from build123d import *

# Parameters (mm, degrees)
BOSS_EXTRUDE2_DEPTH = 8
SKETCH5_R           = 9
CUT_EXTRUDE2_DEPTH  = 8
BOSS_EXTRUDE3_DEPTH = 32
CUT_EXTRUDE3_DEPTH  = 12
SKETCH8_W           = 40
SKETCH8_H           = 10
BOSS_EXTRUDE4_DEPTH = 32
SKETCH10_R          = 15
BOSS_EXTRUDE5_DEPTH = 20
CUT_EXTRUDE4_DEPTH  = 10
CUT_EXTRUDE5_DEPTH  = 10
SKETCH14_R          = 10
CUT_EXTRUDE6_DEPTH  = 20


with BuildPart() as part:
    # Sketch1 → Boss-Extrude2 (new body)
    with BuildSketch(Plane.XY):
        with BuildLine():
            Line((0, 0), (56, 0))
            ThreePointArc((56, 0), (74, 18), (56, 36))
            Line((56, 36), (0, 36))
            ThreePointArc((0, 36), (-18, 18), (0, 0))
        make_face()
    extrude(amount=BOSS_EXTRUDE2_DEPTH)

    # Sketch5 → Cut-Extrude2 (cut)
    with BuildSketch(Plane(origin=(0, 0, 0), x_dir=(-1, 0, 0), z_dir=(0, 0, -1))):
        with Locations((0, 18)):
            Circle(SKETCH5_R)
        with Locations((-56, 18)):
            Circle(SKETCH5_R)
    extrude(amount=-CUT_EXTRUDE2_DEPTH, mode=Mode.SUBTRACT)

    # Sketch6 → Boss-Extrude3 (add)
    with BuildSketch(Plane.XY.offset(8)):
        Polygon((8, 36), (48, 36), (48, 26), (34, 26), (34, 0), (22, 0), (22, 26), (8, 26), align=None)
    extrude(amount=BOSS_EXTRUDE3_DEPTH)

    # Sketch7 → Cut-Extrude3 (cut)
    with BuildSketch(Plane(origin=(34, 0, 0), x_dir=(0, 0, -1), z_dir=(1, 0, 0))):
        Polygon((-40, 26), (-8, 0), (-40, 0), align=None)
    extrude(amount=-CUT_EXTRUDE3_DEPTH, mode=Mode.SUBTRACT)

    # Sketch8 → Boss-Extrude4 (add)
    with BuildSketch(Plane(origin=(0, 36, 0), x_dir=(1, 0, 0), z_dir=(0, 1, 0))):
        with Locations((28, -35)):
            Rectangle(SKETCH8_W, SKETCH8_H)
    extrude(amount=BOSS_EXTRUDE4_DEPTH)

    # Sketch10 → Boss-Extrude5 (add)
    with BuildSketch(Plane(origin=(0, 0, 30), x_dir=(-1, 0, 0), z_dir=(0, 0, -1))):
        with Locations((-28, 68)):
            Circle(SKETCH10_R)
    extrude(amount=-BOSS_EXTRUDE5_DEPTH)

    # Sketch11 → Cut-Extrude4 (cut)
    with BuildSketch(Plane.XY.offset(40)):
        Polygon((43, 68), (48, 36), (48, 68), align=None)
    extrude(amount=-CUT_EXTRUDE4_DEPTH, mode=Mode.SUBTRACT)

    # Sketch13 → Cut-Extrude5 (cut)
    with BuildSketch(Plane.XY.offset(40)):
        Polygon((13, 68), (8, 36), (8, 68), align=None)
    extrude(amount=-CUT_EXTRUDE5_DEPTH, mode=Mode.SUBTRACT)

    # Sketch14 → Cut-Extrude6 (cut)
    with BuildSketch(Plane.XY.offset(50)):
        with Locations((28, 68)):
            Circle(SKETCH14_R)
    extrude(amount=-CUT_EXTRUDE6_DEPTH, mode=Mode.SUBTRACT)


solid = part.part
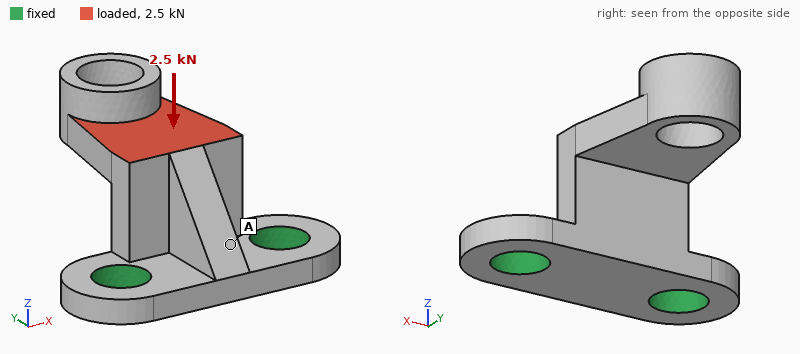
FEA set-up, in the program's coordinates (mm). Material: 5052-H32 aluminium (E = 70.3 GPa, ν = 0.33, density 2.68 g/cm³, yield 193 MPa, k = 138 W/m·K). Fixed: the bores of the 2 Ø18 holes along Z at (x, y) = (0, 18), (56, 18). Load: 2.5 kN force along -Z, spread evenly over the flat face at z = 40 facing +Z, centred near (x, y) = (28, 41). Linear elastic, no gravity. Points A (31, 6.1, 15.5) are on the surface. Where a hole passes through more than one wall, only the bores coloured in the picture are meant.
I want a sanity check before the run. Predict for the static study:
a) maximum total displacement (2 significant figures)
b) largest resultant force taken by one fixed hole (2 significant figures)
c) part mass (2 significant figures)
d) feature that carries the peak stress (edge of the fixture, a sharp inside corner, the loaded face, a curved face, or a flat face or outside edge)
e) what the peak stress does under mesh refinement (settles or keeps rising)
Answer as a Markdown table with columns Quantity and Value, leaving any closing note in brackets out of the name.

| Quantity | Value |
|---|---|
| maximum total displacement | 0.17 mm |
| largest resultant force taken by one fixed hole | 1.4 kN |
| part mass | 140 g |
| feature that carries the peak stress | edge of the fixture |
| what the peak stress does under mesh refinement | keeps rising |
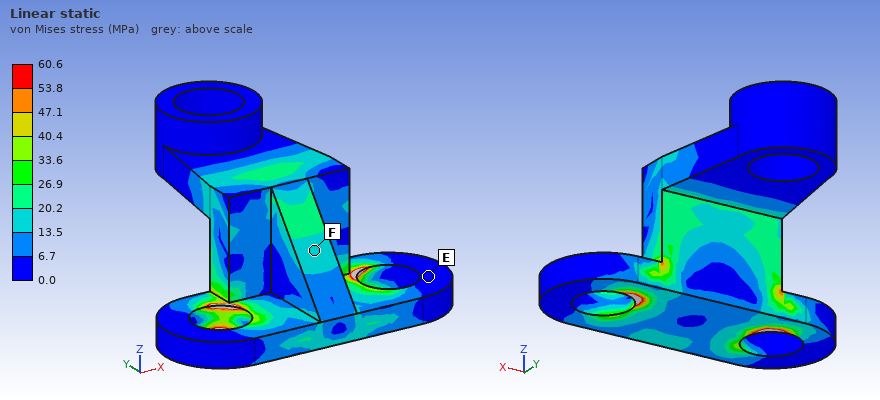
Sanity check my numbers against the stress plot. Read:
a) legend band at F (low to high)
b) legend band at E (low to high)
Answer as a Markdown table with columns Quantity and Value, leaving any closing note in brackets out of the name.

| Quantity | Value |
|---|---|
| legend band at F | 13.5 to 20.2 MPa |
| legend band at E | 0.0 to 6.7 MPa |
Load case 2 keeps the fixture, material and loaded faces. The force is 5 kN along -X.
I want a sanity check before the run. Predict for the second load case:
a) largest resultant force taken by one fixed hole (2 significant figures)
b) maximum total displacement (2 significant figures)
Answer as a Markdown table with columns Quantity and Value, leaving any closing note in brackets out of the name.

| Quantity | Value |
|---|---|
| largest resultant force taken by one fixed hole | 5.5 kN |
| maximum total displacement | 0.17 mm |
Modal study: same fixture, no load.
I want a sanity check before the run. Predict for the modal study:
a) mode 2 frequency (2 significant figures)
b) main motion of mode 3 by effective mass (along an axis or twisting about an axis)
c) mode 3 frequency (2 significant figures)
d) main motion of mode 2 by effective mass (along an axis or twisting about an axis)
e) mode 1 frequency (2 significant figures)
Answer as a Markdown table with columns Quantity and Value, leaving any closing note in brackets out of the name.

| Quantity | Value |
|---|---|
| mode 2 frequency | 3400 Hz |
| main motion of mode 3 by effective mass | along Y |
| mode 3 frequency | 5300 Hz |
| main motion of mode 2 by effective mass | along X |
| mode 1 frequency | 2100 Hz |
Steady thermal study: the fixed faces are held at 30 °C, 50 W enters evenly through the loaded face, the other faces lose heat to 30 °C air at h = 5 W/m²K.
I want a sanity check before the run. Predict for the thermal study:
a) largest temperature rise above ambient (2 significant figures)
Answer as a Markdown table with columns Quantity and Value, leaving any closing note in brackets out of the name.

| Quantity | Value |
|---|---|
| largest temperature rise above ambient | 36 K |
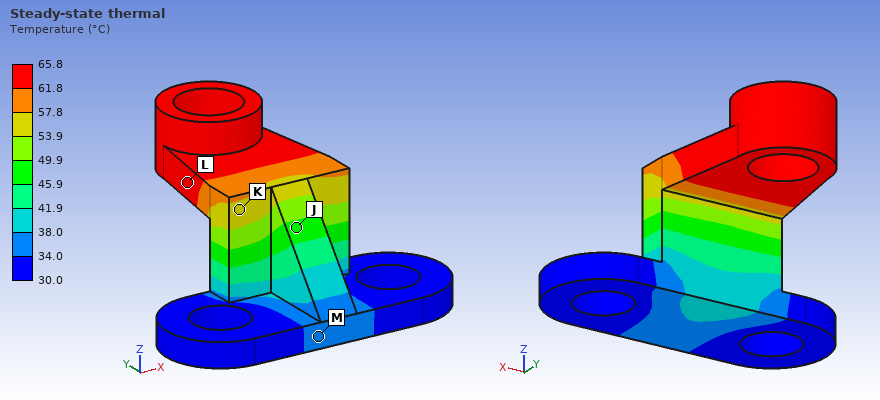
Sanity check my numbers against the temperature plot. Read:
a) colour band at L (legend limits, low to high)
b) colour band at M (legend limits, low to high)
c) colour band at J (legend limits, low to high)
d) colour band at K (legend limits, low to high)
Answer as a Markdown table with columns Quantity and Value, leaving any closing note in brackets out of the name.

| Quantity | Value |
|---|---|
| colour band at L | 61.8 to 65.8 °C |
| colour band at M | 34.0 to 38.0 °C |
| colour band at J | 45.9 to 49.9 °C |
| colour band at K | 53.9 to 57.8 °C |
